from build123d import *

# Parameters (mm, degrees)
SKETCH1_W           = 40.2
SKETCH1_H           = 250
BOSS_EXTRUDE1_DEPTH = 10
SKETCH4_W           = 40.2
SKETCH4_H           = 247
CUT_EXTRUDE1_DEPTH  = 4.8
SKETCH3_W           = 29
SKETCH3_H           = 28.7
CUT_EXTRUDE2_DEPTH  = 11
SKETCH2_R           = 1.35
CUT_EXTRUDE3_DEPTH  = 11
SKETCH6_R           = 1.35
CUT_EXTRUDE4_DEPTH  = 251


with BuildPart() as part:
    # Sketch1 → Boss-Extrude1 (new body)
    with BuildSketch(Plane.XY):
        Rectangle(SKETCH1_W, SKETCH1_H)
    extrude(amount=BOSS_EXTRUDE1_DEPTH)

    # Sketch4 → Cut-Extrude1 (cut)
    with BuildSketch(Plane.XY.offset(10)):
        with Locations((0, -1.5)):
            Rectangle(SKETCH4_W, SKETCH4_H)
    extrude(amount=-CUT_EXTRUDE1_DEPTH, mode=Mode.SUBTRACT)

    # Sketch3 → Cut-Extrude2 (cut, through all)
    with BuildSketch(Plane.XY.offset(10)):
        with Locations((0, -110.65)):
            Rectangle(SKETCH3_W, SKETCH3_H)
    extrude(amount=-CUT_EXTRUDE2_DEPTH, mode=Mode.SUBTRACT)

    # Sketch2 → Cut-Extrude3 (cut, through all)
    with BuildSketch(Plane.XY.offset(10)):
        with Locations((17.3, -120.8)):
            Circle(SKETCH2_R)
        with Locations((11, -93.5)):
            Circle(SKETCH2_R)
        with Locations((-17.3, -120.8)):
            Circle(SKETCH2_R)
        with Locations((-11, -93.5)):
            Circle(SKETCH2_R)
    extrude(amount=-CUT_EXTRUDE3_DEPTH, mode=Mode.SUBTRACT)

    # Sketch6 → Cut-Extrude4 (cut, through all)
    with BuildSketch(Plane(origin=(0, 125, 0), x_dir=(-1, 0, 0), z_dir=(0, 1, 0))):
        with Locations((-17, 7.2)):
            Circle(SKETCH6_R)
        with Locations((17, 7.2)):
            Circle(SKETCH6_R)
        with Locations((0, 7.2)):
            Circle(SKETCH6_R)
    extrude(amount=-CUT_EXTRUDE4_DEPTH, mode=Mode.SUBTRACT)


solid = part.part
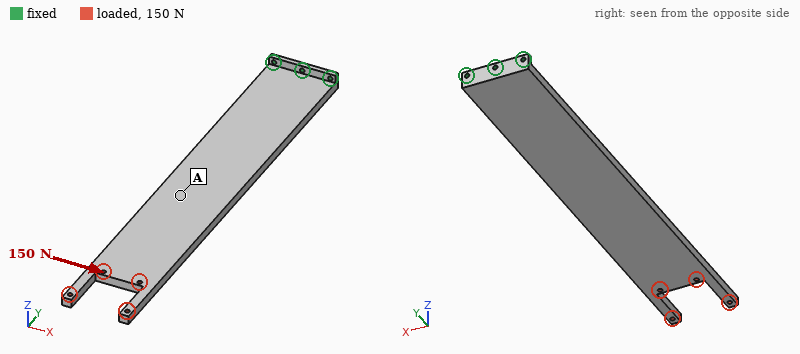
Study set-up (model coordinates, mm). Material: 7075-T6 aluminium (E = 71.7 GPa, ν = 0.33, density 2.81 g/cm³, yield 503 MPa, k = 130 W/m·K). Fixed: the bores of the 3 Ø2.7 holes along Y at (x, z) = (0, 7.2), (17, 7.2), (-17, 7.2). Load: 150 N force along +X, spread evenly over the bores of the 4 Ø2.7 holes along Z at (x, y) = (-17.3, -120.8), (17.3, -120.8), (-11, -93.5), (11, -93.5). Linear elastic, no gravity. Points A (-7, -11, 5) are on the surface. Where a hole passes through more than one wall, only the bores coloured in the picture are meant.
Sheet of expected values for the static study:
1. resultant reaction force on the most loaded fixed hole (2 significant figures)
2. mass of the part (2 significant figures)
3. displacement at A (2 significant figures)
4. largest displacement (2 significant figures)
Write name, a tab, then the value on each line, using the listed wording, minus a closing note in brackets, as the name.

resultant reaction force on the most loaded fixed hole	1.0 kN
mass of the part	140 g
displacement at A	0.22 mm
largest displacement	0.58 mm
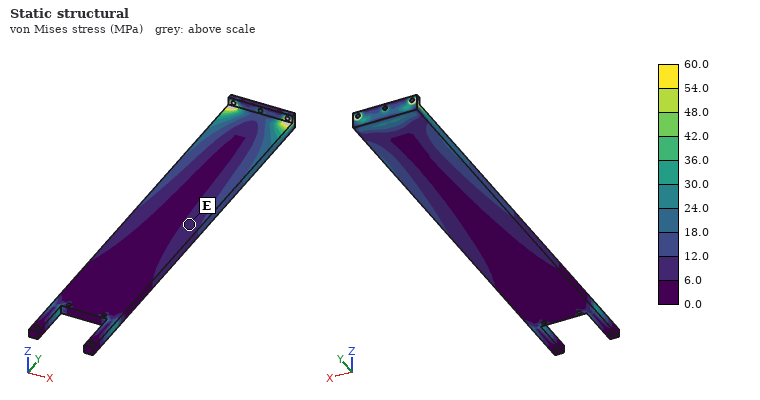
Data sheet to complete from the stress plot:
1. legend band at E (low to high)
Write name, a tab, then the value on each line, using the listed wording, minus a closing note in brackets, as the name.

legend band at E	6.0 to 12.0 MPa
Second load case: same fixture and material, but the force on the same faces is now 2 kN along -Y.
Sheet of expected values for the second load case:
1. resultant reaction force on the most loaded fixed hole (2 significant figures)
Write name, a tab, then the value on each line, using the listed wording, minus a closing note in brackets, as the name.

resultant reaction force on the most loaded fixed hole	710 N
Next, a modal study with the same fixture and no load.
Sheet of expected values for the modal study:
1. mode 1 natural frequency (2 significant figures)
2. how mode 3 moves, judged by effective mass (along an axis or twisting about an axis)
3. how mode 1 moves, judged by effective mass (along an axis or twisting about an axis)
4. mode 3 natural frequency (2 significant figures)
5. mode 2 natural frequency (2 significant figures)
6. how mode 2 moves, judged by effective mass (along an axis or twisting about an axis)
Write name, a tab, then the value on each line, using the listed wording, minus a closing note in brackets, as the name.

mode 1 natural frequency	71 Hz
how mode 3 moves, judged by effective mass	along X
how mode 1 moves, judged by effective mass	along Z
mode 3 natural frequency	480 Hz
mode 2 natural frequency	450 Hz
how mode 2 moves, judged by effective mass	along Z
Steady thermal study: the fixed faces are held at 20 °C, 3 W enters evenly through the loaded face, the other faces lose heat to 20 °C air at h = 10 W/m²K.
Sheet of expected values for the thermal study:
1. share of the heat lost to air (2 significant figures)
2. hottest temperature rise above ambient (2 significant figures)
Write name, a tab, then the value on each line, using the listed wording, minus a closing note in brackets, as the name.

share of the heat lost to air	54 %
hottest temperature rise above ambient	20 K
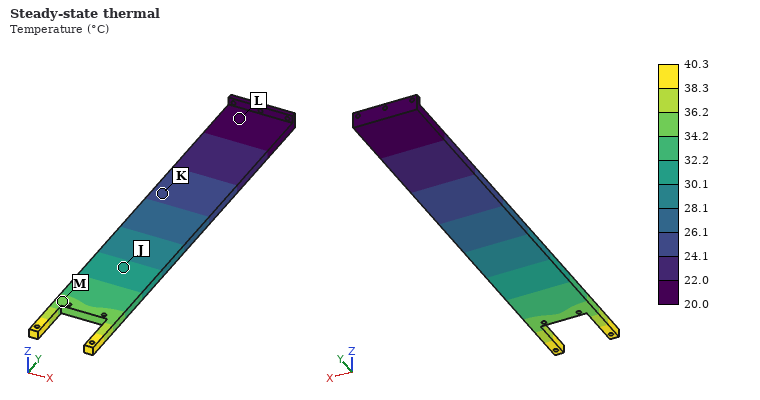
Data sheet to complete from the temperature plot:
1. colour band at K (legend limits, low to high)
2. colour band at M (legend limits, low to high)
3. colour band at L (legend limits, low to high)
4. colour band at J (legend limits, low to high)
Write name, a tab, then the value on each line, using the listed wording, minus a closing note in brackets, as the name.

colour band at K	24.1 to 26.1 °C
colour band at M	34.2 to 36.2 °C
colour band at L	20.0 to 22.0 °C
colour band at J	30.1 to 32.2 °C
